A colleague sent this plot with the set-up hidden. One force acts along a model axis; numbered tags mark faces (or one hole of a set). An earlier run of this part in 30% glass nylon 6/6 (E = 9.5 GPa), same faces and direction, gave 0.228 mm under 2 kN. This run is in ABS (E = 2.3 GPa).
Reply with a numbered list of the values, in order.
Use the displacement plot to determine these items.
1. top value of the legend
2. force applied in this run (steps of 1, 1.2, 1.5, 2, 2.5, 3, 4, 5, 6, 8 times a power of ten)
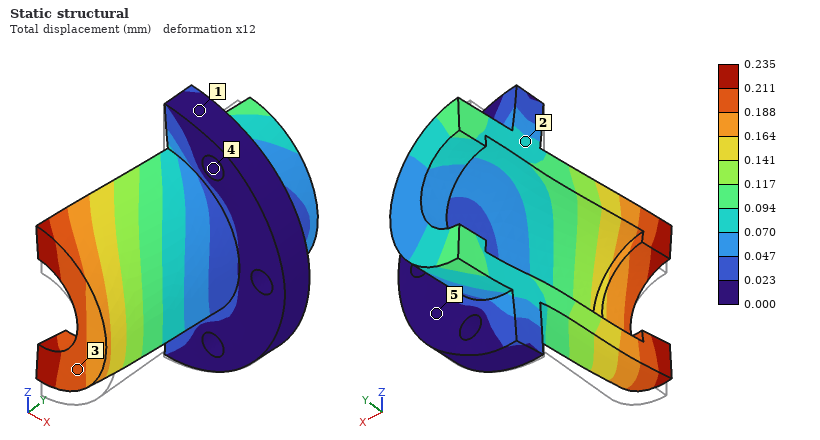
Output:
1. 0.235 mm
2. 500 N
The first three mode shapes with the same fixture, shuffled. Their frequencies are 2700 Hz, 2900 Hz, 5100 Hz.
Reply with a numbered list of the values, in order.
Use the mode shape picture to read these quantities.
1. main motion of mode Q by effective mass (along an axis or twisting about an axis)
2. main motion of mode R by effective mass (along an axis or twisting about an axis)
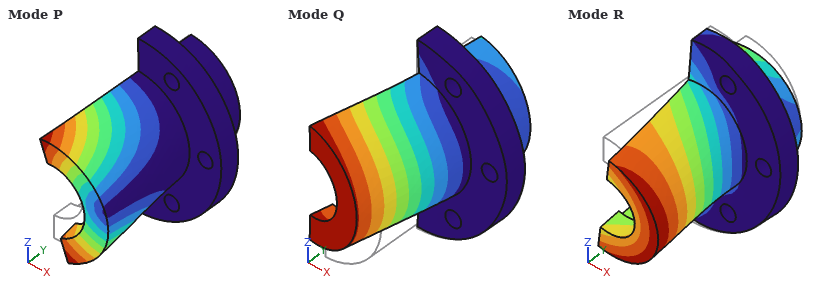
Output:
1. along X
2. along Z
